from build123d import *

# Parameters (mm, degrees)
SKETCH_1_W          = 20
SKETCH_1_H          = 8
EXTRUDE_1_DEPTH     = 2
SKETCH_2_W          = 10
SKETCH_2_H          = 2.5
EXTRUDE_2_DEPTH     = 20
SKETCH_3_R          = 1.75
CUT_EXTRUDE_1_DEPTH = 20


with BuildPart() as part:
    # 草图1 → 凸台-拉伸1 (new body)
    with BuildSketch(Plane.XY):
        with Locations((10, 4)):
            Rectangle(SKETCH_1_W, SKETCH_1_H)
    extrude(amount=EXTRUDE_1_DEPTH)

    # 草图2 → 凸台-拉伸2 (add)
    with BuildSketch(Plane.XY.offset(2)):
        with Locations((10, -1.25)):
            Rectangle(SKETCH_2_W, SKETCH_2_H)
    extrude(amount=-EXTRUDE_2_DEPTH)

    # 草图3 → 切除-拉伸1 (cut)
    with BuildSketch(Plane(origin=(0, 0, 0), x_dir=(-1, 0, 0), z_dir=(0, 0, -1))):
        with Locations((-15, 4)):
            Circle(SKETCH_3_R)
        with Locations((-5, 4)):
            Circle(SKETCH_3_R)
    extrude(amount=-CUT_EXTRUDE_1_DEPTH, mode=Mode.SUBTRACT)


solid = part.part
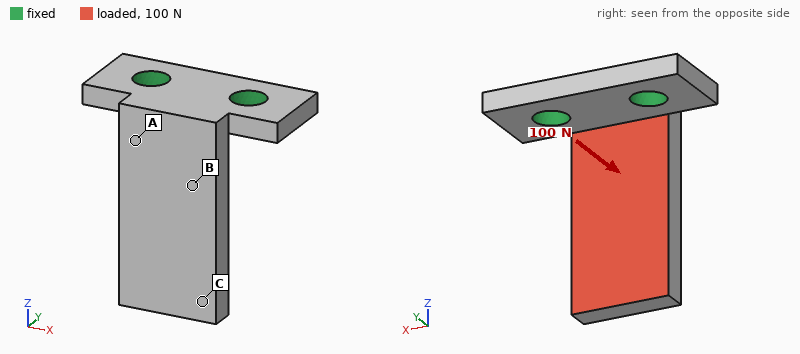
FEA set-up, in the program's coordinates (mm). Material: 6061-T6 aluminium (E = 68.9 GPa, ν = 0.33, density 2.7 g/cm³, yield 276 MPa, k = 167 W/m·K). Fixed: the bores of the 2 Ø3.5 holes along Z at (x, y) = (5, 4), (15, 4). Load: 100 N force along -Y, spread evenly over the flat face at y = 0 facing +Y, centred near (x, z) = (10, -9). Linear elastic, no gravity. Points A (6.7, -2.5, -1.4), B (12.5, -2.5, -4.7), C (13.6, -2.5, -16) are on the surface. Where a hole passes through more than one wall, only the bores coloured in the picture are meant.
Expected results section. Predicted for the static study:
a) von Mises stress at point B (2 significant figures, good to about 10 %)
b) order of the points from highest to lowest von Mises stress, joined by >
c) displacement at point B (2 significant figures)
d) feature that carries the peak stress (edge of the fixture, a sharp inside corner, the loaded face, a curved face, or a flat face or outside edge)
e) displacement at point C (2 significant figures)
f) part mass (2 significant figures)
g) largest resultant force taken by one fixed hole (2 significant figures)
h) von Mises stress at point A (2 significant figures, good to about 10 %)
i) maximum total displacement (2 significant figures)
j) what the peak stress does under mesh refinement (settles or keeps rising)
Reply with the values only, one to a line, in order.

45 MPa
A > B > C
0.059 mm
a sharp inside corner
0.19 mm
2.1 g
56 N
70 MPa
0.22 mm
keeps rising
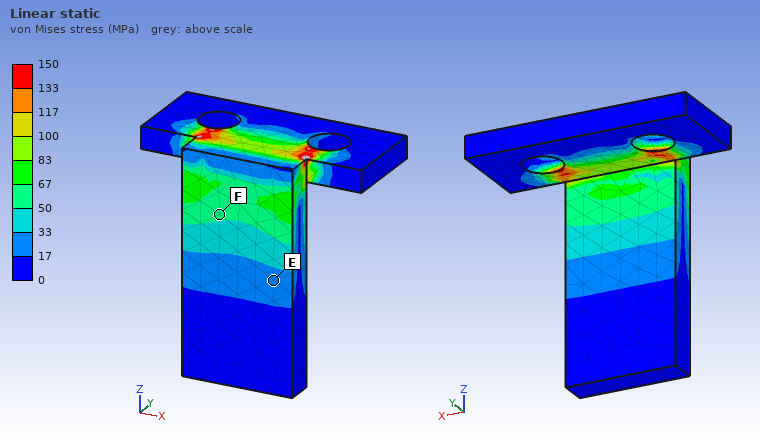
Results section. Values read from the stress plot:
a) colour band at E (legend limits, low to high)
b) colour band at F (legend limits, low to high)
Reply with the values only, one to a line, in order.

17 to 33 MPa
50 to 67 MPa
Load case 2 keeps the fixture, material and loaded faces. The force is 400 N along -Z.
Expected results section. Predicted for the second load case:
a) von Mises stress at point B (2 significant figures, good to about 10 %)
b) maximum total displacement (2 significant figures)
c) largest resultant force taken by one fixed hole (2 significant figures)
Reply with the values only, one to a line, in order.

23 MPa
19 µm
200 N
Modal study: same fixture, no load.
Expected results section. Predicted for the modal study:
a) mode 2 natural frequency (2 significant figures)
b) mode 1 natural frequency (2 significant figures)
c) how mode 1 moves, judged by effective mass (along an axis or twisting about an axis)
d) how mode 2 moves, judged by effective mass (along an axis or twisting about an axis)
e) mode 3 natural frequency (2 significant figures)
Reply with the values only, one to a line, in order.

9700 Hz
3800 Hz
along Y
along X
20 kHz
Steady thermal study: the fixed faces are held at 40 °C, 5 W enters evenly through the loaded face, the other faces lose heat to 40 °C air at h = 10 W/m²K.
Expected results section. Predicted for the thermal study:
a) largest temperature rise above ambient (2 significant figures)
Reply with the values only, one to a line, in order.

17 K
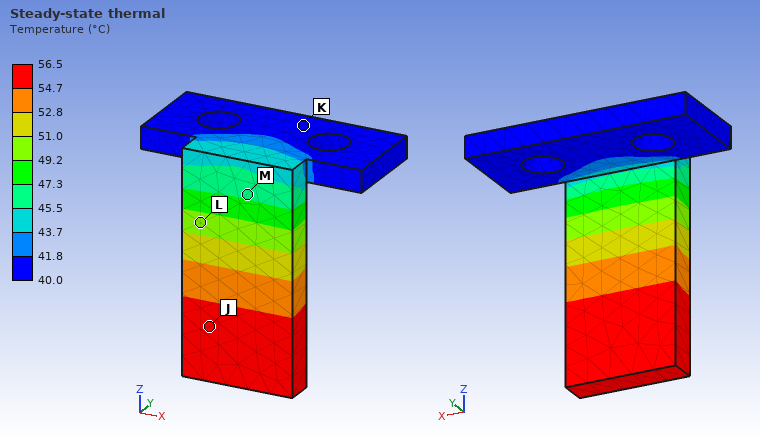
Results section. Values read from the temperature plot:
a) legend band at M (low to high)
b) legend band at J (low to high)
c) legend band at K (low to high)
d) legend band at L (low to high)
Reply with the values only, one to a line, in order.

45.5 to 47.3 °C
54.7 to 56.5 °C
40.0 to 41.8 °C
49.2 to 51.0 °C
